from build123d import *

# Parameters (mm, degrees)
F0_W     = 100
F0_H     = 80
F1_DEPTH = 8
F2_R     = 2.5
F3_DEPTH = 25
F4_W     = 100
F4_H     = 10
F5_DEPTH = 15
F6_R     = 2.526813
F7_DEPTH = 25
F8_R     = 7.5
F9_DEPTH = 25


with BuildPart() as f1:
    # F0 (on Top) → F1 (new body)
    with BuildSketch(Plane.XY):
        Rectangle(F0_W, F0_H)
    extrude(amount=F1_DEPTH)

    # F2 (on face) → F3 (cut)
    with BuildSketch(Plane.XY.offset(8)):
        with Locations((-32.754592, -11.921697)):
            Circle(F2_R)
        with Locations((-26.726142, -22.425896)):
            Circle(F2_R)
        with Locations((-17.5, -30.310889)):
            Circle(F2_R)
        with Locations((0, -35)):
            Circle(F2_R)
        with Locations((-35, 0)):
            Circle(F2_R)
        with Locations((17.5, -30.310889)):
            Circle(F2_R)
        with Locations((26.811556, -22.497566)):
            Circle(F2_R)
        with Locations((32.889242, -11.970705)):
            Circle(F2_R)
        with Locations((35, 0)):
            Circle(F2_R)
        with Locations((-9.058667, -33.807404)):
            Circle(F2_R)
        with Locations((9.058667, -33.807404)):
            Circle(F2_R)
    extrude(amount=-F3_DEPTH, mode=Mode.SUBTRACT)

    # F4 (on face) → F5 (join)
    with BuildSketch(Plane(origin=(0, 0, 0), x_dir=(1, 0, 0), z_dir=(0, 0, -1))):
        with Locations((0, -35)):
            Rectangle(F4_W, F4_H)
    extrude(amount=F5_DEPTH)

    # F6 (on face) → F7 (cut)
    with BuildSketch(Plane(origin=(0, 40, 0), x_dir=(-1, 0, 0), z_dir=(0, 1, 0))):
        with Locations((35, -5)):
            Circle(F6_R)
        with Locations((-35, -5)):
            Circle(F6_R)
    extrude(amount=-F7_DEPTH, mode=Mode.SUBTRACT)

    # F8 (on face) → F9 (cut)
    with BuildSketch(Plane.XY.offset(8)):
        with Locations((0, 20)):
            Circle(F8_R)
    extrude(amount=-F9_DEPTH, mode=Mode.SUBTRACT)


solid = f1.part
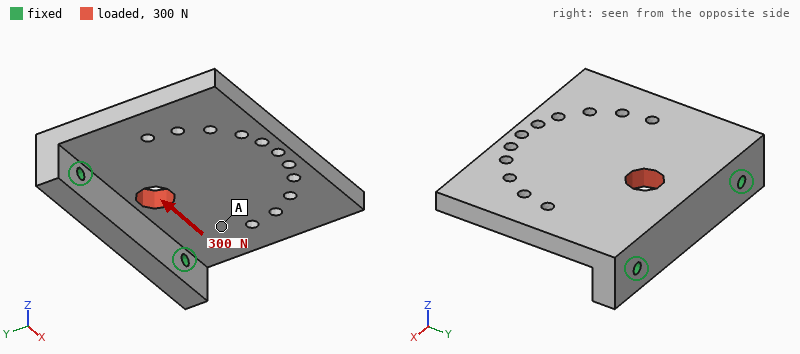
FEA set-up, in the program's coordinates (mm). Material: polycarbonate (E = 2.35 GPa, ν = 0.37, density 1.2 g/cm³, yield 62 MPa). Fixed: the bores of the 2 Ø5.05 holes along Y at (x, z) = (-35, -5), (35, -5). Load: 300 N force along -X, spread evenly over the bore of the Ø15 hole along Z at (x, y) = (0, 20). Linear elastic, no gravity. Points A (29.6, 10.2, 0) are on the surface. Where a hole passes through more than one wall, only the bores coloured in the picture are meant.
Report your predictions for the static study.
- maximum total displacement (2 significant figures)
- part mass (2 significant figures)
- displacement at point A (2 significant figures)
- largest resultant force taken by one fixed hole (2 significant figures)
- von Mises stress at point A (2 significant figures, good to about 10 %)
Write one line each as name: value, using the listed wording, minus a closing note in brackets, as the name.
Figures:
maximum total displacement: 33 µm
part mass: 91 g
displacement at point A: 19 µm
largest resultant force taken by one fixed hole: 170 N
von Mises stress at point A: 0.31 MPa
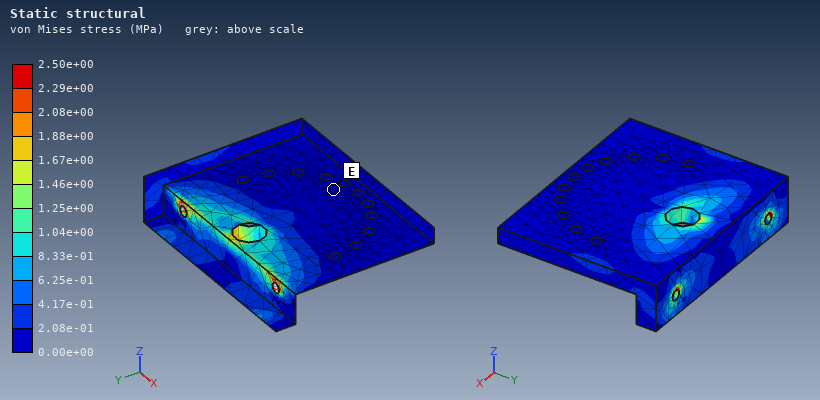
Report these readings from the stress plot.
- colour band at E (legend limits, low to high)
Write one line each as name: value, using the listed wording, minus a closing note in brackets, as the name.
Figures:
colour band at E: 0.00e+00 to 2.08e-01 MPa
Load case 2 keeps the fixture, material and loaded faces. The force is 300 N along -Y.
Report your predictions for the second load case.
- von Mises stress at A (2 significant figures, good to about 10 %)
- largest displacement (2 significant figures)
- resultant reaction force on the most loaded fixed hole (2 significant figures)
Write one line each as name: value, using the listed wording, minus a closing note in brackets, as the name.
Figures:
von Mises stress at A: 0.54 MPa
largest displacement: 0.15 mm
resultant reaction force on the most loaded fixed hole: 150 N
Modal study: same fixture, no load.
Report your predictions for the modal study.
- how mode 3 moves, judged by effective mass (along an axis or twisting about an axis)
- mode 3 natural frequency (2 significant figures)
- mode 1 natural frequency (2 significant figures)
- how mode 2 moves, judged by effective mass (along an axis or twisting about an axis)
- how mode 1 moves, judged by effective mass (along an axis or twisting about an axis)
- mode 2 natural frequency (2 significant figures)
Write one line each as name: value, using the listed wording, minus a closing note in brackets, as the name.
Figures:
how mode 3 moves, judged by effective mass: along X
mode 3 natural frequency: 1400 Hz
mode 1 natural frequency: 280 Hz
how mode 2 moves, judged by effective mass: twisting about Y
how mode 1 moves, judged by effective mass: along Z
mode 2 natural frequency: 580 Hz
